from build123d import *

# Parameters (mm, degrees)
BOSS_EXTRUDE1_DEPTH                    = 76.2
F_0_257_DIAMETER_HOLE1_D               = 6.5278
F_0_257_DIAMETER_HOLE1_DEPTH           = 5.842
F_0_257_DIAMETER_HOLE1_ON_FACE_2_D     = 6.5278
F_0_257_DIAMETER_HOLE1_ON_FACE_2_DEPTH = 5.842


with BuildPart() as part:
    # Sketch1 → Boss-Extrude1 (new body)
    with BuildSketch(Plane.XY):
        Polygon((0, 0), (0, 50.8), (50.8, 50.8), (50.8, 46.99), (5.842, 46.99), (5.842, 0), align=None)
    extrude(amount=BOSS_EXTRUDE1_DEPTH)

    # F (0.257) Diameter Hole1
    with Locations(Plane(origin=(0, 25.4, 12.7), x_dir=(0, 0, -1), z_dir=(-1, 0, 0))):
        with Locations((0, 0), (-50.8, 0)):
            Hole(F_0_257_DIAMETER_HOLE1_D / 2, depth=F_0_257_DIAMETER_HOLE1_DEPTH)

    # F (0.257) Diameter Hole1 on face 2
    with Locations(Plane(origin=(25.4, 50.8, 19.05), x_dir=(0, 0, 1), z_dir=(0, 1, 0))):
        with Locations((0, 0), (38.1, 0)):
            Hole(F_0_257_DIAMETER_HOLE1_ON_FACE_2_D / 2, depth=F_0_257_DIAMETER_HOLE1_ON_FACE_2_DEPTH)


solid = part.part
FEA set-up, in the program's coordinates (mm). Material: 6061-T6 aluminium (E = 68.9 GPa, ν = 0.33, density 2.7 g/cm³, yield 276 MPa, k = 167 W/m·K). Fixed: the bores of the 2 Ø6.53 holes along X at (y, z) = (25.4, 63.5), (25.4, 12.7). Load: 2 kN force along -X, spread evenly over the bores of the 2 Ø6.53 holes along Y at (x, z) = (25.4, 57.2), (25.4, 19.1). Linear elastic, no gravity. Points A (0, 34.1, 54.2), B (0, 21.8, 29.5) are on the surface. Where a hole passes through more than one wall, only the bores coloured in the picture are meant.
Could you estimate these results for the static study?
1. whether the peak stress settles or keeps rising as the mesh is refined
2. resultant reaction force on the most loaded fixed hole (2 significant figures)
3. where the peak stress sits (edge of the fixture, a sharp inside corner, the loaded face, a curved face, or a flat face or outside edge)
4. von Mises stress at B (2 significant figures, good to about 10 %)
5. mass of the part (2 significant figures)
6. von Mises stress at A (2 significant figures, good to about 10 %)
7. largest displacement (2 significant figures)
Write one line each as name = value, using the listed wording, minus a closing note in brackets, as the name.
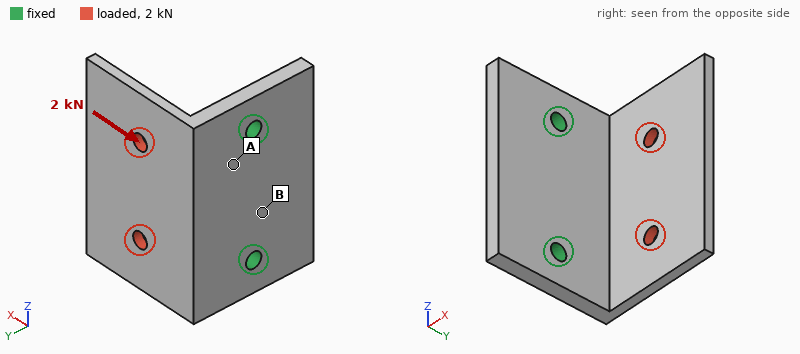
whether the peak stress settles or keeps rising as the mesh is refined = keeps rising
resultant reaction force on the most loaded fixed hole = 1.0 kN
where the peak stress sits = edge of the fixture
von Mises stress at B = 25 MPa
mass of the part = 95 g
von Mises stress at A = 56 MPa
largest displacement = 0.34 mm
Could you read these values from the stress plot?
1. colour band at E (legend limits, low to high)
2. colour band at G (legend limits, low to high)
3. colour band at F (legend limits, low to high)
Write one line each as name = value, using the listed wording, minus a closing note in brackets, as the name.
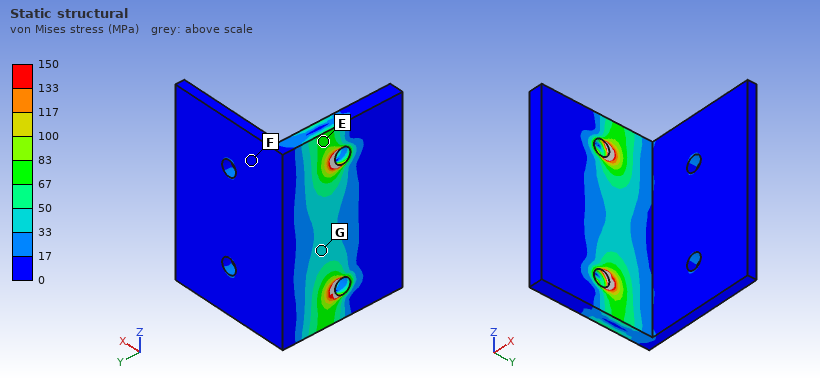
colour band at E = 67 to 83 MPa
colour band at G = 33 to 50 MPa
colour band at F = 0 to 17 MPa
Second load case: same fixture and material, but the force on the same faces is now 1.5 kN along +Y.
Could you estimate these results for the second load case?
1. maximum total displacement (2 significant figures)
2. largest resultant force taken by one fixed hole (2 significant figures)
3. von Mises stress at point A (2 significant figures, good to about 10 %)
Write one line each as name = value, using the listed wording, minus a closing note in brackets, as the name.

maximum total displacement = 0.94 mm
largest resultant force taken by one fixed hole = 760 N
von Mises stress at point A = 62 MPa
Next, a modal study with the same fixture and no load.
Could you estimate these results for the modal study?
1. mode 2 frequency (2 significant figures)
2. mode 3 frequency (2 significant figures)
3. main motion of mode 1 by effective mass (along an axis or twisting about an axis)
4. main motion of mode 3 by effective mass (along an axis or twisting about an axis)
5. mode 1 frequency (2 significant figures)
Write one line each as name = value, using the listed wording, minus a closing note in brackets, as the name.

mode 2 frequency = 2100 Hz
mode 3 frequency = 3300 Hz
main motion of mode 1 by effective mass = along Y
main motion of mode 3 by effective mass = along Z
mode 1 frequency = 1100 Hz
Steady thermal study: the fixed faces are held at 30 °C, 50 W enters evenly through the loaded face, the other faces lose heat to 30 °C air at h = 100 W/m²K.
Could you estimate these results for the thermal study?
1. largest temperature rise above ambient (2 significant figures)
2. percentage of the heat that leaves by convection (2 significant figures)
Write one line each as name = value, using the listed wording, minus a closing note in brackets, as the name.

largest temperature rise above ambient = 33 K
percentage of the heat that leaves by convection = 41 %
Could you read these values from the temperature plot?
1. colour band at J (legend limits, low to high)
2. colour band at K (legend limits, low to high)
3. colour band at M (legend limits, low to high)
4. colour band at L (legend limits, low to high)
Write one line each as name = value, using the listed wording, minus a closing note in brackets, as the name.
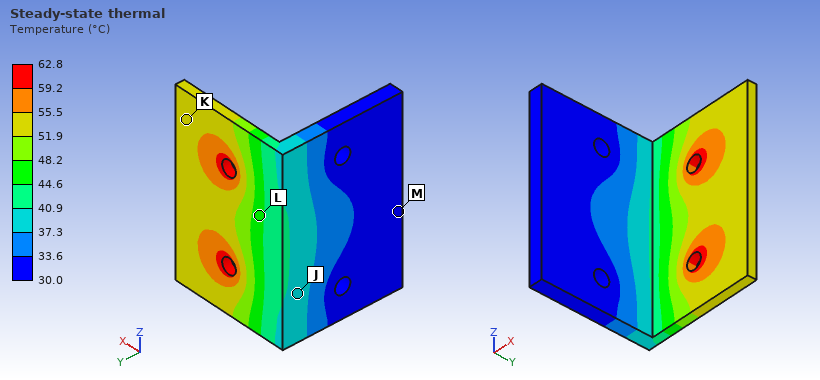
colour band at J = 37.3 to 40.9 °C
colour band at K = 51.9 to 55.5 °C
colour band at M = 30.0 to 33.6 °C
colour band at L = 44.6 to 48.2 °C
